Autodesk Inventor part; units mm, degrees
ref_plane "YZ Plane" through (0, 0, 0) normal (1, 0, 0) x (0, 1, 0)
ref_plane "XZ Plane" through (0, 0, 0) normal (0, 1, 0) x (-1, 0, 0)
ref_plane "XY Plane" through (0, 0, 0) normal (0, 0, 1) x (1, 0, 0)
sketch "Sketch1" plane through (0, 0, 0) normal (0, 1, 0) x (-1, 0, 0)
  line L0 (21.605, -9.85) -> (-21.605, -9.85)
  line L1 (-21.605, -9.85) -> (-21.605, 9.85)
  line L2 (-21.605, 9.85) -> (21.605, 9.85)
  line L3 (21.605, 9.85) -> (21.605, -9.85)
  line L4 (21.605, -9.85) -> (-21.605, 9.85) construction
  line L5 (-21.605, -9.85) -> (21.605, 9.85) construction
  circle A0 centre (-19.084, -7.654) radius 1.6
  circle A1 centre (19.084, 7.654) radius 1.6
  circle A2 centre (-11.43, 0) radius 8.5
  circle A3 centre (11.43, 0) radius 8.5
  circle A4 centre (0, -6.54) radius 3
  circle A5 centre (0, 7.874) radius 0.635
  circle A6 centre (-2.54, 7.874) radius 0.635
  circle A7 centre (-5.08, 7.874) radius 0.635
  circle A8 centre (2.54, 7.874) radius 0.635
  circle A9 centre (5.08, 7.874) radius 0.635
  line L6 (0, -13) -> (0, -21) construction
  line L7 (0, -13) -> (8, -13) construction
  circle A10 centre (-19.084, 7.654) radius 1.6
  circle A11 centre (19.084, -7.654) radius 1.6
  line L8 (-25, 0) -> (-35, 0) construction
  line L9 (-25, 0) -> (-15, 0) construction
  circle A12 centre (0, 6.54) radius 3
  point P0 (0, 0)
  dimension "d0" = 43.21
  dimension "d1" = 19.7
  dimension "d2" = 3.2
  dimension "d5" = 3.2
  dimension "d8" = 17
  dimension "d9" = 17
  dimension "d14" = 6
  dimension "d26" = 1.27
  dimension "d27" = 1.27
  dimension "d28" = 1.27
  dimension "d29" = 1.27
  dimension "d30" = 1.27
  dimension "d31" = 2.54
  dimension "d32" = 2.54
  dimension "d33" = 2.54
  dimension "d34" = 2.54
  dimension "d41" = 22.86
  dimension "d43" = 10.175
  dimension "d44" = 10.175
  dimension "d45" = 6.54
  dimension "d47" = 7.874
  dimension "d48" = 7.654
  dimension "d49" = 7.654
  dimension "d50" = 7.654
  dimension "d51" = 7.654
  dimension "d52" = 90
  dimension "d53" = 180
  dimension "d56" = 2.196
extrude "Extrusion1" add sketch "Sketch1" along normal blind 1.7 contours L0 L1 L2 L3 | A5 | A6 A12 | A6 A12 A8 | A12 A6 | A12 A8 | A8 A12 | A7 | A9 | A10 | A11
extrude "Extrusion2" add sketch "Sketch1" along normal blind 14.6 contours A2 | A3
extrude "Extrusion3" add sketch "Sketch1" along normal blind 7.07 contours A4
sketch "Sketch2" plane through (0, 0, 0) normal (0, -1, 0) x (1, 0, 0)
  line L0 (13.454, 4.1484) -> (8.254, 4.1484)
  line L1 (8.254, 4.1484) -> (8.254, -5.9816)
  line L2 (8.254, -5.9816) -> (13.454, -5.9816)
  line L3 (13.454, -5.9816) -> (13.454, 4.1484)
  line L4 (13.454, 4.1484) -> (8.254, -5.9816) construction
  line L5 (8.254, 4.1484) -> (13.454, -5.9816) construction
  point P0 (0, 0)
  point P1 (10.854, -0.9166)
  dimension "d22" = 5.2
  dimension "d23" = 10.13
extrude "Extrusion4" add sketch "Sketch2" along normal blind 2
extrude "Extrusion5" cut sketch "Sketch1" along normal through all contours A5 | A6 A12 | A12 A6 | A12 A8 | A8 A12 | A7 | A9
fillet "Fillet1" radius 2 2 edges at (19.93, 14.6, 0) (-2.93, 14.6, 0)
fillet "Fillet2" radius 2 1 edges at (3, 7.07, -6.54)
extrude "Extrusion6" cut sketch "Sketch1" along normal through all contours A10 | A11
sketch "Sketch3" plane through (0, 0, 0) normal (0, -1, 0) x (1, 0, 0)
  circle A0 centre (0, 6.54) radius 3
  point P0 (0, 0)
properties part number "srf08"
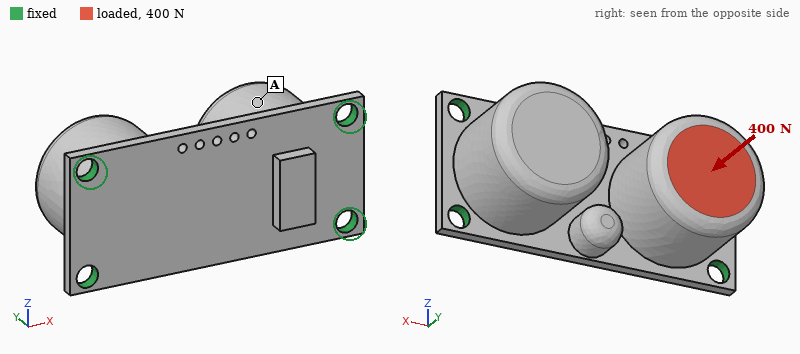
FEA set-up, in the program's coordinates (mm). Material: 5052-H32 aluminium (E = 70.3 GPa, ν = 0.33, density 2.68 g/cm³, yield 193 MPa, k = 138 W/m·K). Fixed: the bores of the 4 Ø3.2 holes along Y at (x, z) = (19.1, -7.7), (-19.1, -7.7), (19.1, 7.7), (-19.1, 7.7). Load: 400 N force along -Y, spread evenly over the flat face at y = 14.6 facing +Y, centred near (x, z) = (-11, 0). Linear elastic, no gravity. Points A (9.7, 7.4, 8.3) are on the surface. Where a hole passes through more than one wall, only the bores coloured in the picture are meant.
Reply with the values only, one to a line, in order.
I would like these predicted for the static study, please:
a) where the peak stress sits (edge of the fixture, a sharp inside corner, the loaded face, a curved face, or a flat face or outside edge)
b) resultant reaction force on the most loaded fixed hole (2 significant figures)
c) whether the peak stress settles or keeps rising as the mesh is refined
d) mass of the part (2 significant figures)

edge of the fixture
170 N
keeps rising
20 g
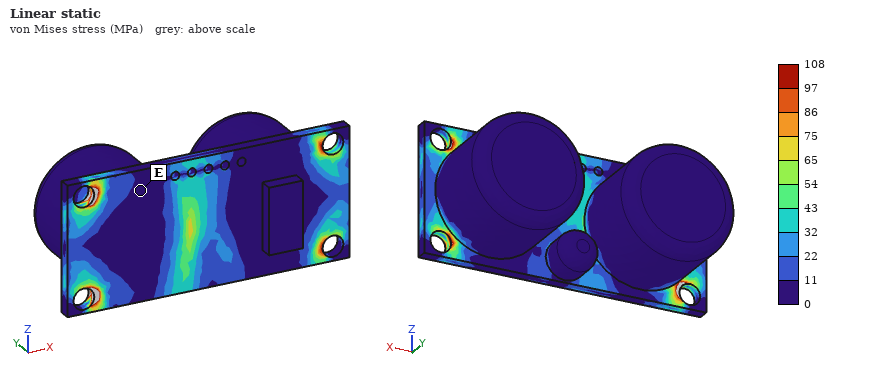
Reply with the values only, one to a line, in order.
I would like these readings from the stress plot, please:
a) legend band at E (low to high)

0 to 11 MPa
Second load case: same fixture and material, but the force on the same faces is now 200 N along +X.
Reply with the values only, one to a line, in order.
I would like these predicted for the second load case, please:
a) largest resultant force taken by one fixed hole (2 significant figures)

96 N
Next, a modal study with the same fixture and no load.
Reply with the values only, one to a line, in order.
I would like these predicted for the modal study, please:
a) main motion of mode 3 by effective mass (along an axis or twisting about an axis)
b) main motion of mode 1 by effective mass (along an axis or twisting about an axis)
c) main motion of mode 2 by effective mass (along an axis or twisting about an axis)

along Z
along Y
along X
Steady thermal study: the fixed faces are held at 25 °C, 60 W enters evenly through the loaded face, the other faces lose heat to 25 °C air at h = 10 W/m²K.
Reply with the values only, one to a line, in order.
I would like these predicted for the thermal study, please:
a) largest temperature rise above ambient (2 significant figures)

70 K
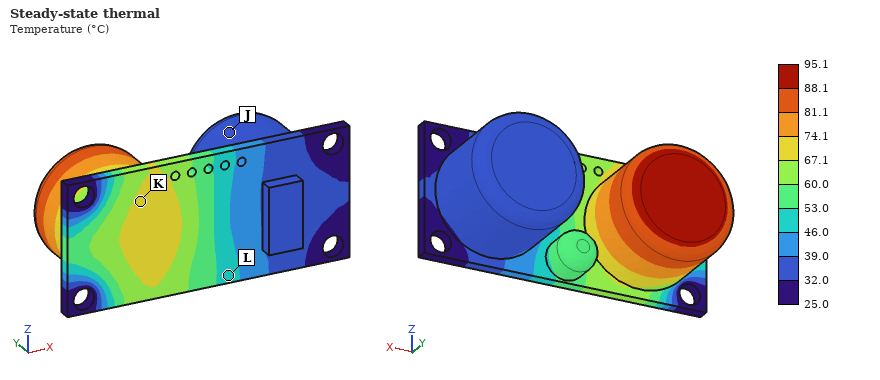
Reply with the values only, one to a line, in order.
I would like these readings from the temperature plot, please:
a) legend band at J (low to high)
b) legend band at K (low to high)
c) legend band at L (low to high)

32.0 to 39.0 °C
67.1 to 74.1 °C
46.0 to 53.0 °C
